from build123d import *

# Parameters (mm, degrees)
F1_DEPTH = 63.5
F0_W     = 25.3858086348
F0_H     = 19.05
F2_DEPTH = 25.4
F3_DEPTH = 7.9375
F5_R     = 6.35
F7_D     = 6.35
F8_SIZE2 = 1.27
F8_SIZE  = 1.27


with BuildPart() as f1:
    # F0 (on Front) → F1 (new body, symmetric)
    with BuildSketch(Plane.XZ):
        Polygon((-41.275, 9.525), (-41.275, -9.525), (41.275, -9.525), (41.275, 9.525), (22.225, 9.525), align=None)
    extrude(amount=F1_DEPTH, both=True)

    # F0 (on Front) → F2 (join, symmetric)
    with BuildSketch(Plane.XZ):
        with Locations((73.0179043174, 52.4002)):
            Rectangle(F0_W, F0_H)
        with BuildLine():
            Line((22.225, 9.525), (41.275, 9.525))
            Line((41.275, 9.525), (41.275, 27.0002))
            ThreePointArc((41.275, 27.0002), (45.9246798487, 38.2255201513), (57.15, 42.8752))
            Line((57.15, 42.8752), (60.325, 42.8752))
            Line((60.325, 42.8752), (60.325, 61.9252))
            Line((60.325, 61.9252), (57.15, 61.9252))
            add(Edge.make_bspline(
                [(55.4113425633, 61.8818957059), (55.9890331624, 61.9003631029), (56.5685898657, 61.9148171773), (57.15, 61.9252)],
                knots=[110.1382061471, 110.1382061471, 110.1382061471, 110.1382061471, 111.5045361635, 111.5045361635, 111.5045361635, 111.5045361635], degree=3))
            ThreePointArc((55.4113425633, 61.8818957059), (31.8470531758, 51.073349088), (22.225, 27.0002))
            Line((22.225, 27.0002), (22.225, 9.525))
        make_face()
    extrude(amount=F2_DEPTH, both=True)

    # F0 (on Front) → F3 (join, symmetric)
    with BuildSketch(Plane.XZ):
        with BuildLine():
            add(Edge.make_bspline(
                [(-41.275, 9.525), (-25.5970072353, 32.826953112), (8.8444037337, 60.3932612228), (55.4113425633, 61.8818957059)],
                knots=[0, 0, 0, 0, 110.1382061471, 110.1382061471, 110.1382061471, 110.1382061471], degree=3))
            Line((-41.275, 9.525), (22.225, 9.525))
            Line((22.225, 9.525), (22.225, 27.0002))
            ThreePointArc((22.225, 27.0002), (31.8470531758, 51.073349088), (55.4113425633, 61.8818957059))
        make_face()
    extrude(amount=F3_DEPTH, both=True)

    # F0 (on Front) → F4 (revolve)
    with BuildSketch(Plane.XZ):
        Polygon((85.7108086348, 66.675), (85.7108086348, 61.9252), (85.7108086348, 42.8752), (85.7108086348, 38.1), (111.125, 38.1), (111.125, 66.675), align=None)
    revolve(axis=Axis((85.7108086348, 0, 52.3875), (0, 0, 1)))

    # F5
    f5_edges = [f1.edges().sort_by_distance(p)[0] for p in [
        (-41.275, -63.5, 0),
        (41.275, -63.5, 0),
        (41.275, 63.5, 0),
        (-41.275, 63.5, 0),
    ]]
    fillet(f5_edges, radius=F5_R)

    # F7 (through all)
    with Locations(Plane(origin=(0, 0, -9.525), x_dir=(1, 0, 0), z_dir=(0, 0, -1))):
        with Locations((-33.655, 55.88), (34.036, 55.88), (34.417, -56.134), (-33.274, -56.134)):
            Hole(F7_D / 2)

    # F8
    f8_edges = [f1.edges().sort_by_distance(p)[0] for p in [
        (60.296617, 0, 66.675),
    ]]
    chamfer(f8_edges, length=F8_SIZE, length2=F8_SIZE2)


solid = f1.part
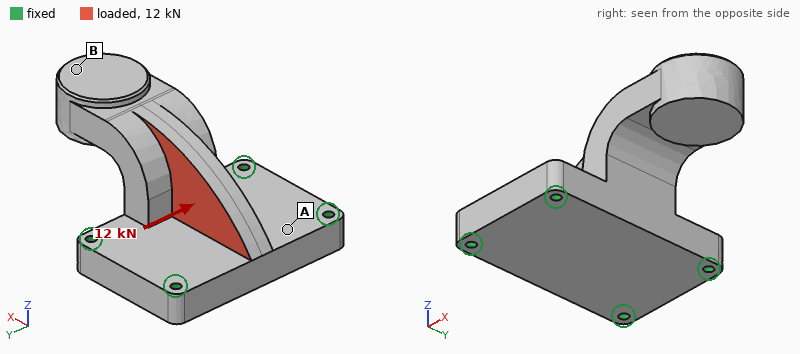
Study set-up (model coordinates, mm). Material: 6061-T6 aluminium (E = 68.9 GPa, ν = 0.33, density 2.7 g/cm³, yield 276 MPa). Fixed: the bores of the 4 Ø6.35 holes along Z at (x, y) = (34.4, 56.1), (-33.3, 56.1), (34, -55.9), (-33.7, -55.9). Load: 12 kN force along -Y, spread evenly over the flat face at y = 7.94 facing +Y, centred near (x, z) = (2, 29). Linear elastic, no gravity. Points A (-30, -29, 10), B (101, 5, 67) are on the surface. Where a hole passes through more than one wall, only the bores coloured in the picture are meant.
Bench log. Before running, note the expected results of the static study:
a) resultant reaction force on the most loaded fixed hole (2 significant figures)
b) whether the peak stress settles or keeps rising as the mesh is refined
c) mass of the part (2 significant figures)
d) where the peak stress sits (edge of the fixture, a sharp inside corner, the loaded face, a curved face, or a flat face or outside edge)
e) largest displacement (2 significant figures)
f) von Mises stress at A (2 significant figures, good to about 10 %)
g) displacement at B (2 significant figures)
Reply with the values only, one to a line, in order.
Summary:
4.3 kN
keeps rising
950 g
edge of the fixture
63 µm
12 MPa
16 µm
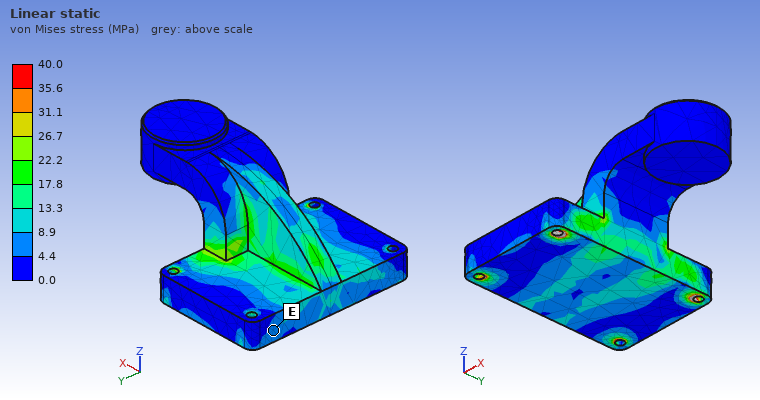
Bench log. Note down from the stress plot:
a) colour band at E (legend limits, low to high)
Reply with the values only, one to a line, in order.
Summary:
4.4 to 8.9 MPa
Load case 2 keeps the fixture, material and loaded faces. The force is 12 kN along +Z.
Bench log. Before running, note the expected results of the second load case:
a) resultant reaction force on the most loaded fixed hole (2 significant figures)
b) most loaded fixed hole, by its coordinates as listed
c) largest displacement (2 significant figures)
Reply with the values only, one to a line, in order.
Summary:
3.9 kN
(34.4, 56.1)
52 µm
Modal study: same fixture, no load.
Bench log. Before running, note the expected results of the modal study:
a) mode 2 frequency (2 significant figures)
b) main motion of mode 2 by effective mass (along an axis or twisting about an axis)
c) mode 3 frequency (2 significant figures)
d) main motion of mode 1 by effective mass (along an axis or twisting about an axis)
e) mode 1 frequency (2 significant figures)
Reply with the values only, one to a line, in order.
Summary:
1800 Hz
along Y
3700 Hz
along Z
1500 Hz
